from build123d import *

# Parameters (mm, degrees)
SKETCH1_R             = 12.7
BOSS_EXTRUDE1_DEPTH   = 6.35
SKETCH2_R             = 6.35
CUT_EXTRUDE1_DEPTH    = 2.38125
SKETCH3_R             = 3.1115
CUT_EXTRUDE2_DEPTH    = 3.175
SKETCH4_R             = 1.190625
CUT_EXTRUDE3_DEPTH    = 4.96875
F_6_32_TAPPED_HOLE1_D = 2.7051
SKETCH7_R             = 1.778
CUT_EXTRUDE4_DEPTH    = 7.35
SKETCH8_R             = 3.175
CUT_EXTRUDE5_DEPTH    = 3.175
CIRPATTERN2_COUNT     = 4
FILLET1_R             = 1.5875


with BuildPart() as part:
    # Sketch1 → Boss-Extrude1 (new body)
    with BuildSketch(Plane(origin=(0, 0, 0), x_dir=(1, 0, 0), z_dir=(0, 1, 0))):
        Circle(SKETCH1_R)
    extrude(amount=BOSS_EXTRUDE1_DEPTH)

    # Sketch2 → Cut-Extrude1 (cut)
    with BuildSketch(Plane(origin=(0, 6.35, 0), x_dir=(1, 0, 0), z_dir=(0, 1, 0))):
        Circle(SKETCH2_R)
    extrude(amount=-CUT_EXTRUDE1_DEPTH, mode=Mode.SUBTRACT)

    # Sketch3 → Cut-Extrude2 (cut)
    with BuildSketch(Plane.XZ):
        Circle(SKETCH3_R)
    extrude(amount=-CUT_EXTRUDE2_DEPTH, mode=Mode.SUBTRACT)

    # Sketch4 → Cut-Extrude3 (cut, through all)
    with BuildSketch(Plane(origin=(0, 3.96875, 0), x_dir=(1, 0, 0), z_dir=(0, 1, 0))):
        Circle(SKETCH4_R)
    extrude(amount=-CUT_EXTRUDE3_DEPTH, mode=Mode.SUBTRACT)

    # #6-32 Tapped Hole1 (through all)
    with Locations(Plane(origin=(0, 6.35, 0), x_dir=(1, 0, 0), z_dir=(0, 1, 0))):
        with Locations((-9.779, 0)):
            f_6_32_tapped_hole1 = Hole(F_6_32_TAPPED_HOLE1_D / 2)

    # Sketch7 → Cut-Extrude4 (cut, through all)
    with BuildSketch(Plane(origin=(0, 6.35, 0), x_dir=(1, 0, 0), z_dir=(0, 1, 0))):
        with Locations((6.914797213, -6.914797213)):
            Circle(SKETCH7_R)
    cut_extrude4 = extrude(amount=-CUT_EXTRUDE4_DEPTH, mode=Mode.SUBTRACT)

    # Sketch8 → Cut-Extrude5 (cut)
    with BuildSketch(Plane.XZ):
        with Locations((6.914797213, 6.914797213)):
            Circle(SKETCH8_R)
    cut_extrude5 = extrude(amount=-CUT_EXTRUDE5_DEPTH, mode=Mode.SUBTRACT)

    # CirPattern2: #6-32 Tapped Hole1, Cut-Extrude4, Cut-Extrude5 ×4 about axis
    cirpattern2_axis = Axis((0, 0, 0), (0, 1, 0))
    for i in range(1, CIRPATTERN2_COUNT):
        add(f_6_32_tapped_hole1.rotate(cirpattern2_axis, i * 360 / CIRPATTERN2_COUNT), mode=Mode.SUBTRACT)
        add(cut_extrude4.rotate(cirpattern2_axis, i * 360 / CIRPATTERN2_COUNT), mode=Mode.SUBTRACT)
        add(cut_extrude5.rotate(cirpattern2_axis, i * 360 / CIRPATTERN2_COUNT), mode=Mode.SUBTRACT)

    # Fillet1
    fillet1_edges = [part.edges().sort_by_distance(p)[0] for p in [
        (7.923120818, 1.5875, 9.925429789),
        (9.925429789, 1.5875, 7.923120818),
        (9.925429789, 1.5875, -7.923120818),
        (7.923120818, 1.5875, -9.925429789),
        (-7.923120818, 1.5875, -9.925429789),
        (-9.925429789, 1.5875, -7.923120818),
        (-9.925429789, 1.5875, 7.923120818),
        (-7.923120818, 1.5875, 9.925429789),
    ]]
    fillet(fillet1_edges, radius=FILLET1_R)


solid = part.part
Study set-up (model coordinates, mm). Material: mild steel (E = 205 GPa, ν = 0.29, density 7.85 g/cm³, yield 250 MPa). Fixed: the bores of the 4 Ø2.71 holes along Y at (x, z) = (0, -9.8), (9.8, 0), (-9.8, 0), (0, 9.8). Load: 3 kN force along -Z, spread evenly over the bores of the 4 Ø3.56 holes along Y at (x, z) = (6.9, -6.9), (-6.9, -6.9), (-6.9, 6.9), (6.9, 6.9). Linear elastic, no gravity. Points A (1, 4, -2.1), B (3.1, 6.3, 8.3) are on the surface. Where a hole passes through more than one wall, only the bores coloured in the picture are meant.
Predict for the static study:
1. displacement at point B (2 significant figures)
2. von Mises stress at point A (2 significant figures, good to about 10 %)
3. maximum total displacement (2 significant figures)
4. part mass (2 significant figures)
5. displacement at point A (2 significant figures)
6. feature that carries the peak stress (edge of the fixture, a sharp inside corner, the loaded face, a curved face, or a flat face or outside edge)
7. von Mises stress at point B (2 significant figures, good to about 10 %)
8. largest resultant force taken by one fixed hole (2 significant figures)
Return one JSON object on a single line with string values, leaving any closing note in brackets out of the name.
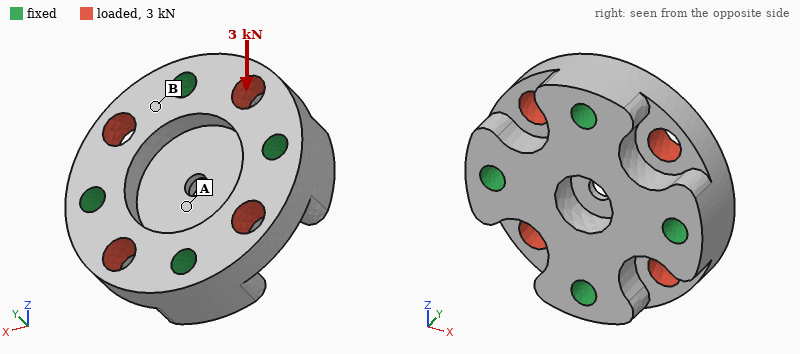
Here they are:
{"displacement at point B": "0.47 µm", "von Mises stress at point A": "11 MPa", "maximum total displacement": "1.7 µm", "part mass": "16 g", "displacement at point A": "0.34 µm", "feature that carries the peak stress": "the loaded face", "von Mises stress at point B": "23 MPa", "largest resultant force taken by one fixed hole": "910 N"}
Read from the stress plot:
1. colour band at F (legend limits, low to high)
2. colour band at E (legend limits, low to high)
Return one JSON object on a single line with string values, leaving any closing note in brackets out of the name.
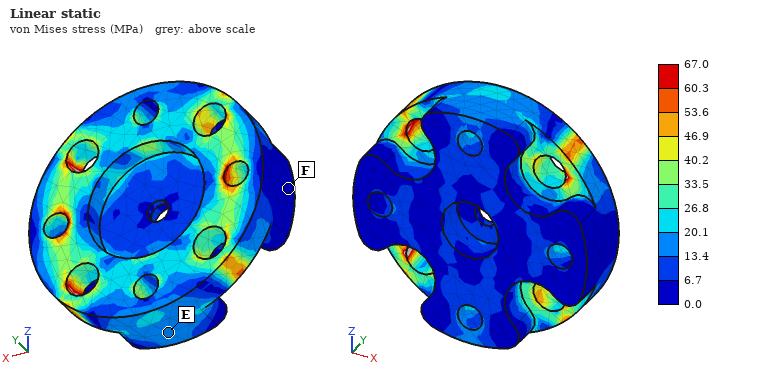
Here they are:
{"colour band at F": "0.0 to 6.7 MPa", "colour band at E": "13.4 to 20.1 MPa"}
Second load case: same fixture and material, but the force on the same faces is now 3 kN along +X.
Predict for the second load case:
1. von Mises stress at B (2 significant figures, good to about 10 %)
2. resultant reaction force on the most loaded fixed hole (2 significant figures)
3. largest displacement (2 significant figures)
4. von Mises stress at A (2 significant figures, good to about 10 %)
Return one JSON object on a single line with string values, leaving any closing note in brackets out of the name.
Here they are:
{"von Mises stress at B": "33 MPa", "resultant reaction force on the most loaded fixed hole": "910 N", "largest displacement": "1.7 µm", "von Mises stress at A": "5.7 MPa"}
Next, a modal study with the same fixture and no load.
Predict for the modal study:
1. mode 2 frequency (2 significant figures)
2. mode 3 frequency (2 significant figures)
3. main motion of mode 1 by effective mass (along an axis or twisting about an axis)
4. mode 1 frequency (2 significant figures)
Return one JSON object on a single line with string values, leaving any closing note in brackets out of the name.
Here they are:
{"mode 2 frequency": "94 kHz", "mode 3 frequency": "96 kHz", "main motion of mode 1 by effective mass": "along Y", "mode 1 frequency": "90 kHz"}
